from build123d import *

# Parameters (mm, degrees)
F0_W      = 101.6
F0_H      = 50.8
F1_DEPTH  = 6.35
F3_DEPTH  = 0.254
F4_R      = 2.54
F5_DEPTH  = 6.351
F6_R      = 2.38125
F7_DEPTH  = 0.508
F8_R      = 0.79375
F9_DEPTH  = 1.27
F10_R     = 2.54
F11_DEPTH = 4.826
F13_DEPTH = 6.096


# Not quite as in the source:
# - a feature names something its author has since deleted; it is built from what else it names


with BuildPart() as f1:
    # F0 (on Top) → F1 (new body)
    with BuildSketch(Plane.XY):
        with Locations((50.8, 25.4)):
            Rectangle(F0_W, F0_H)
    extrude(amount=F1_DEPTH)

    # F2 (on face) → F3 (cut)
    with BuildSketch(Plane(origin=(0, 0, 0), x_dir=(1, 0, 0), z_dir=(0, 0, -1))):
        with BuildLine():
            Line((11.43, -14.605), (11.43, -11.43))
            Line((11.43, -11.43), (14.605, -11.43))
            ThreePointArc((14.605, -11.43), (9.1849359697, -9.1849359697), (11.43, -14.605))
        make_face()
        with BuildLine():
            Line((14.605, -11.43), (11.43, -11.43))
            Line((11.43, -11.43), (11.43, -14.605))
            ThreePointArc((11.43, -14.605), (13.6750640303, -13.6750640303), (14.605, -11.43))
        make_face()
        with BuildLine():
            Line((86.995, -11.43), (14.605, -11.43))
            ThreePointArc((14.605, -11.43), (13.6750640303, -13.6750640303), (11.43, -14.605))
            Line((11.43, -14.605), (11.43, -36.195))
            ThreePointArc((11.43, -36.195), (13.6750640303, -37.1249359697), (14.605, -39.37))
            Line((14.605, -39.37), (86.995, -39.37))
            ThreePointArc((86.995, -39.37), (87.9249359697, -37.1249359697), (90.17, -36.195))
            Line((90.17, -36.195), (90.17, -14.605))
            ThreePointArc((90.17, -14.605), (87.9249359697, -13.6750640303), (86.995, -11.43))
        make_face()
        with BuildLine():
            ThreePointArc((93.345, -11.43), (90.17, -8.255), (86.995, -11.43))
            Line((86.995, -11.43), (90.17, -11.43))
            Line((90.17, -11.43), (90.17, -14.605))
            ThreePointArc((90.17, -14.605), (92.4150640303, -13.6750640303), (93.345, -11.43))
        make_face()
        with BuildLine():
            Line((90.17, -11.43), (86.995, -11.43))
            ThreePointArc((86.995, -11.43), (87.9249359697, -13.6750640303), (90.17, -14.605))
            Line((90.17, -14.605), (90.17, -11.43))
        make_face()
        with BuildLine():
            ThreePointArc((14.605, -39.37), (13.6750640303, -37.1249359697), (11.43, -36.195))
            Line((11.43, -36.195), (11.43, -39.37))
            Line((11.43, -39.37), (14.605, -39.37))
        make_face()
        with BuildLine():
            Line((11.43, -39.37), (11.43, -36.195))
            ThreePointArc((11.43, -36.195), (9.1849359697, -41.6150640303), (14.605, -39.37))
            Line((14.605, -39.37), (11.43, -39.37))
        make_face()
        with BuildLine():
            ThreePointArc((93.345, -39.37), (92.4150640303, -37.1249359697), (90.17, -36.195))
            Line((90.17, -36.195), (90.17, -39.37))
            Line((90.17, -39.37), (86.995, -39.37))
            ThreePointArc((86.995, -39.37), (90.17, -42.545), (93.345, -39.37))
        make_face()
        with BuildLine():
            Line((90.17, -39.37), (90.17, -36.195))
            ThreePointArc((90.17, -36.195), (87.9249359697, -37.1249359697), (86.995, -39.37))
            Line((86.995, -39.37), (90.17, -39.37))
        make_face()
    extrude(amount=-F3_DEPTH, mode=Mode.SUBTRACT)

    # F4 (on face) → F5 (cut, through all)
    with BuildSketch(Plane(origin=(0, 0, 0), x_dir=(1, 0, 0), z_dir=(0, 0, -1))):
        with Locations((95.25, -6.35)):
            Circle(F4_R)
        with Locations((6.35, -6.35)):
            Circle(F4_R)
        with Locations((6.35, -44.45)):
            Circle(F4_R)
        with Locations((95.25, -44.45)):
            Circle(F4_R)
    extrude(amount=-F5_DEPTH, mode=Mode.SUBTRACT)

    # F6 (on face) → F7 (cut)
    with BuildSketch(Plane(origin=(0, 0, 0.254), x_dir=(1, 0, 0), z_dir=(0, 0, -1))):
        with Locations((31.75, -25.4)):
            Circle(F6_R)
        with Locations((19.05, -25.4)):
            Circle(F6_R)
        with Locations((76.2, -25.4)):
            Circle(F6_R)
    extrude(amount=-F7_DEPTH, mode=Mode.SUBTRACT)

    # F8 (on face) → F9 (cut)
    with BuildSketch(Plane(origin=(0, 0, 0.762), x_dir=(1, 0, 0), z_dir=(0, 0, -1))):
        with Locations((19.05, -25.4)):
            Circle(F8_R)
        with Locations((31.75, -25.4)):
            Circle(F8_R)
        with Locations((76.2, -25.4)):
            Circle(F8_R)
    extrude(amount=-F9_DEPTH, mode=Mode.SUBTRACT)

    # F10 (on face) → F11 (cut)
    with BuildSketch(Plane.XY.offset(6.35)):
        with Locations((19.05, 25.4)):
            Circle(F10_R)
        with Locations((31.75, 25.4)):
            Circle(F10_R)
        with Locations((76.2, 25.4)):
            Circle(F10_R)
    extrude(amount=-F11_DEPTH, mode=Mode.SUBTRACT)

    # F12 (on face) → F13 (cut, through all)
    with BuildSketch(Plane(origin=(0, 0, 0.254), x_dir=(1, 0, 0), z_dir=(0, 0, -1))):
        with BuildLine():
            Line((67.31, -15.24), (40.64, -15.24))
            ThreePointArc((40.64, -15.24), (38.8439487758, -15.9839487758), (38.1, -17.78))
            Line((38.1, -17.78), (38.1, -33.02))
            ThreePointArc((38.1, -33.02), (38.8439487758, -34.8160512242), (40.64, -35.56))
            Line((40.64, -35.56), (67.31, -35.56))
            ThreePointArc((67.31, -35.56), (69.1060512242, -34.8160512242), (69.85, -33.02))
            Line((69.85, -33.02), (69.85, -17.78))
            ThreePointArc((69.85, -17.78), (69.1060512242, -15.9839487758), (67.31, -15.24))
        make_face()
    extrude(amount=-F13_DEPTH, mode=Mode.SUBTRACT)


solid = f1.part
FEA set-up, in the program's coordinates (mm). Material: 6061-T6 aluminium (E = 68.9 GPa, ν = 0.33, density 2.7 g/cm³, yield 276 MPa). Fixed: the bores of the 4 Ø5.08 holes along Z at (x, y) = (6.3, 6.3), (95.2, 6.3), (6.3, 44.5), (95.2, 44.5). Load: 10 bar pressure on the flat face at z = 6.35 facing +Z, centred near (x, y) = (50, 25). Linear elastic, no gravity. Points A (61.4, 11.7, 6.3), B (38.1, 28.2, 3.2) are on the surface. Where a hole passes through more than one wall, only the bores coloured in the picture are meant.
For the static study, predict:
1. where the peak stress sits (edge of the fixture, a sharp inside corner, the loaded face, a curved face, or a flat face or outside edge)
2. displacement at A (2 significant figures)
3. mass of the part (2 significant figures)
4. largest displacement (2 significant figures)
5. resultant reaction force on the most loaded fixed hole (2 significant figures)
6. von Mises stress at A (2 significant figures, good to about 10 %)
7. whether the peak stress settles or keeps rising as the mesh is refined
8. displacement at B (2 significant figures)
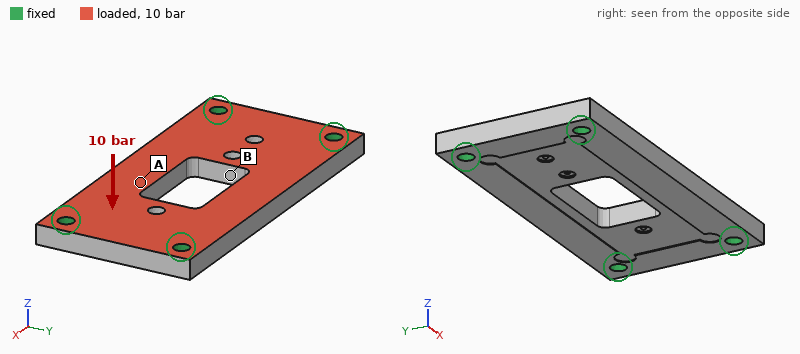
edge of the fixture
0.11 mm
74 g
0.13 mm
1.1 kN
42 MPa
keeps rising
0.11 mm
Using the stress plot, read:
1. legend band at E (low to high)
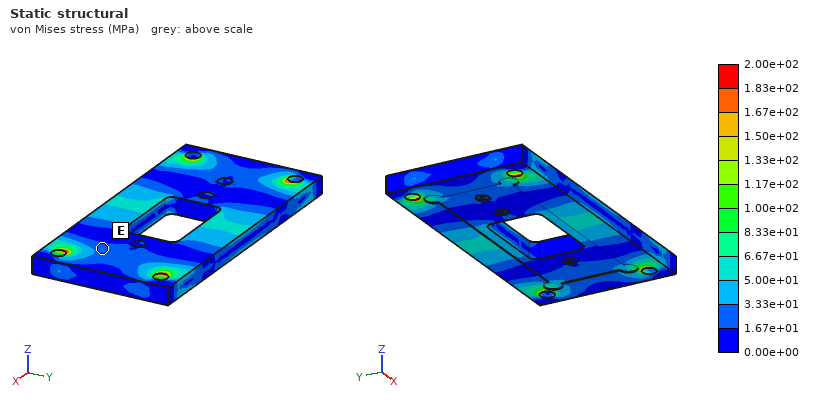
1.67e+01 to 3.33e+01 MPa
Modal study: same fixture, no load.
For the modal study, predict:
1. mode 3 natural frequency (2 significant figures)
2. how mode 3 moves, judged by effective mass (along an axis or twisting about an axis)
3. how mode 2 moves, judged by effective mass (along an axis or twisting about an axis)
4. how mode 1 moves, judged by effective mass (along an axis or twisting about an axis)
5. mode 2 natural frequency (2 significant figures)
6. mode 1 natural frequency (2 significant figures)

9600 Hz
twisting about Y
twisting about X
along Z
5600 Hz
4100 Hz
